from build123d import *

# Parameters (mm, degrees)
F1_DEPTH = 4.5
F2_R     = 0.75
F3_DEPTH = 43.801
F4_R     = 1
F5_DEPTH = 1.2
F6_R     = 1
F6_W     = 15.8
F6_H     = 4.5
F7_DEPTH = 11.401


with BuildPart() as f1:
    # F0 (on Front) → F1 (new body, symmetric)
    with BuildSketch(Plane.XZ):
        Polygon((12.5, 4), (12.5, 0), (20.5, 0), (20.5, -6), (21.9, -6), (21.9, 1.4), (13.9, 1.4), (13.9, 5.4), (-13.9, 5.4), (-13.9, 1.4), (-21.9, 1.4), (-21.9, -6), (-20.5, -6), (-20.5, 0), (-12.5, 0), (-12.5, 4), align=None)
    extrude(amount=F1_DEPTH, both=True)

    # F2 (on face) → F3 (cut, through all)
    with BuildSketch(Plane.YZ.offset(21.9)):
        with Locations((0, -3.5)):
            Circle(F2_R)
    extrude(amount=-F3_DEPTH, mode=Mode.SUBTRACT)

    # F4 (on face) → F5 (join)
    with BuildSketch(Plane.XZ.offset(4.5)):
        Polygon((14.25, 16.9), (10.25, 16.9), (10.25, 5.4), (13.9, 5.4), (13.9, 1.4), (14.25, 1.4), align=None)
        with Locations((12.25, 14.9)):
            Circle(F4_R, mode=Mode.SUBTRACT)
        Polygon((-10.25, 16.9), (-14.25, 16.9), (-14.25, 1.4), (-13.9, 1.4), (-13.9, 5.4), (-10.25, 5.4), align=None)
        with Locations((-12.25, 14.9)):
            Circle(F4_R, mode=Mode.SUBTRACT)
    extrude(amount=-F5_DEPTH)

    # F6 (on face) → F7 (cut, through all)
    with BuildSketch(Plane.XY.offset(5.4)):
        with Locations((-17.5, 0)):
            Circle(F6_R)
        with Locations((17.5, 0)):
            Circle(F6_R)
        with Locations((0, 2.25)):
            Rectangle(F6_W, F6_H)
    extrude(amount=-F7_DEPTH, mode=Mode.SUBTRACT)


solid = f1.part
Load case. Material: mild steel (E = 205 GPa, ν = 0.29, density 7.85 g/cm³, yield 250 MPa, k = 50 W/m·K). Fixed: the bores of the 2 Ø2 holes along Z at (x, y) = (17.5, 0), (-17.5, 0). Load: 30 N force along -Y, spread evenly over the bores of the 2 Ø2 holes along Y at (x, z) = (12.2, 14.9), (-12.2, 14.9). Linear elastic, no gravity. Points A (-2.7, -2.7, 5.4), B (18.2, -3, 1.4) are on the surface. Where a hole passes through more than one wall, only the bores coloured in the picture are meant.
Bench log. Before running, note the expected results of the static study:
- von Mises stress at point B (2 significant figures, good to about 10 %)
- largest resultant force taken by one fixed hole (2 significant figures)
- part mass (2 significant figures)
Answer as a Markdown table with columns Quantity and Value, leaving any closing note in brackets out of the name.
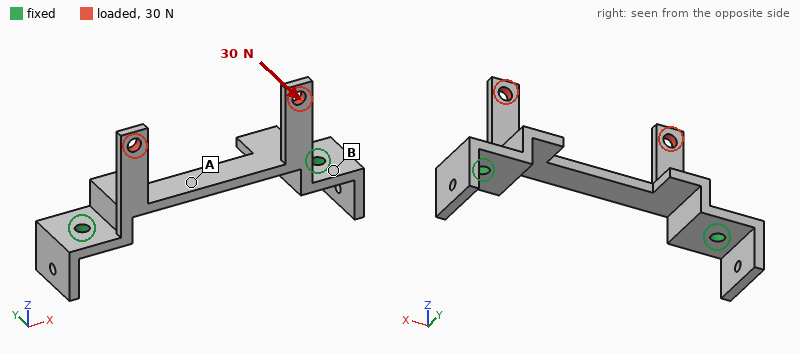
| Quantity | Value |
|---|---|
| von Mises stress at point B | 27 MPa |
| largest resultant force taken by one fixed hole | 15 N |
| part mass | 6.3 g |
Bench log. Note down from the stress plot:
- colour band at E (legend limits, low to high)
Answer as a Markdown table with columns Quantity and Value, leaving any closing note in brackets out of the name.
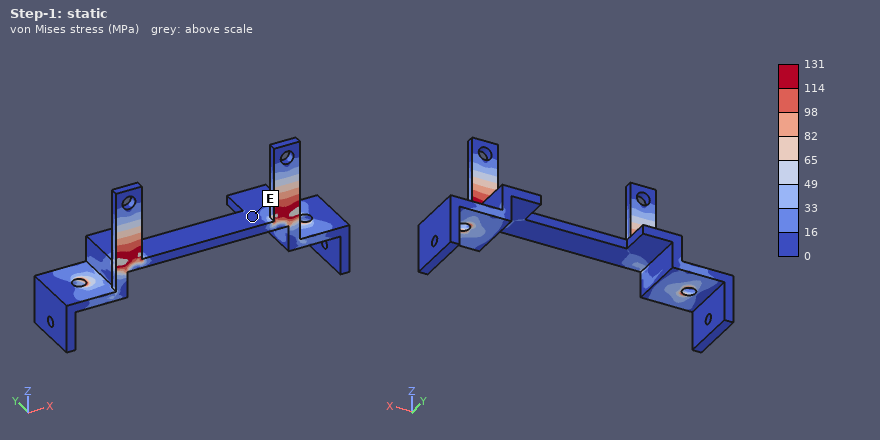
| Quantity | Value |
|---|---|
| colour band at E | 0 to 16 MPa |
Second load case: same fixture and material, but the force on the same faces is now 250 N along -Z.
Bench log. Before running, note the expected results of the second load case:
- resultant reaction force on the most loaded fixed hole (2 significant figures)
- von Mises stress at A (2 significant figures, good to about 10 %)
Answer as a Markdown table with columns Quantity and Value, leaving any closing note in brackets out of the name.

| Quantity | Value |
|---|---|
| resultant reaction force on the most loaded fixed hole | 150 N |
| von Mises stress at A | 19 MPa |
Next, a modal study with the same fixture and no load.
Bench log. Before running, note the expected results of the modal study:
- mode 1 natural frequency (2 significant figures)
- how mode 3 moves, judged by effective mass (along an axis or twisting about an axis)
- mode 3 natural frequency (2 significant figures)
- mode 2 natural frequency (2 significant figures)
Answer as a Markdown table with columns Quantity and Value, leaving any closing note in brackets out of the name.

| Quantity | Value |
|---|---|
| mode 1 natural frequency | 5700 Hz |
| how mode 3 moves, judged by effective mass | along X |
| mode 3 natural frequency | 7400 Hz |
| mode 2 natural frequency | 5900 Hz |
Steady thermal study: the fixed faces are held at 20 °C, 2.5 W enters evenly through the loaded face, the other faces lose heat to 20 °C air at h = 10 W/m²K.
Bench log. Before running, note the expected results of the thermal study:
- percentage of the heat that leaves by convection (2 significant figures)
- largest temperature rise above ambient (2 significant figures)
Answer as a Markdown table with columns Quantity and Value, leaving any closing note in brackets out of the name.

| Quantity | Value |
|---|---|
| percentage of the heat that leaves by convection | 8.6 % |
| largest temperature rise above ambient | 76 K |
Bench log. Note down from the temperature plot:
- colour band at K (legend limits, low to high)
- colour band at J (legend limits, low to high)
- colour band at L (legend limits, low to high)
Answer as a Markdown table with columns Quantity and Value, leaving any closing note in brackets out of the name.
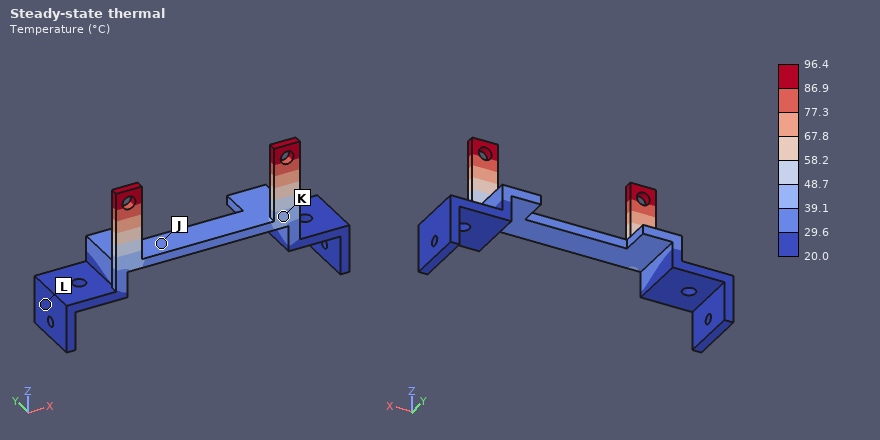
| Quantity | Value |
|---|---|
| colour band at K | 39.1 to 48.7 °C |
| colour band at J | 29.6 to 39.1 °C |
| colour band at L | 20.0 to 29.6 °C |
